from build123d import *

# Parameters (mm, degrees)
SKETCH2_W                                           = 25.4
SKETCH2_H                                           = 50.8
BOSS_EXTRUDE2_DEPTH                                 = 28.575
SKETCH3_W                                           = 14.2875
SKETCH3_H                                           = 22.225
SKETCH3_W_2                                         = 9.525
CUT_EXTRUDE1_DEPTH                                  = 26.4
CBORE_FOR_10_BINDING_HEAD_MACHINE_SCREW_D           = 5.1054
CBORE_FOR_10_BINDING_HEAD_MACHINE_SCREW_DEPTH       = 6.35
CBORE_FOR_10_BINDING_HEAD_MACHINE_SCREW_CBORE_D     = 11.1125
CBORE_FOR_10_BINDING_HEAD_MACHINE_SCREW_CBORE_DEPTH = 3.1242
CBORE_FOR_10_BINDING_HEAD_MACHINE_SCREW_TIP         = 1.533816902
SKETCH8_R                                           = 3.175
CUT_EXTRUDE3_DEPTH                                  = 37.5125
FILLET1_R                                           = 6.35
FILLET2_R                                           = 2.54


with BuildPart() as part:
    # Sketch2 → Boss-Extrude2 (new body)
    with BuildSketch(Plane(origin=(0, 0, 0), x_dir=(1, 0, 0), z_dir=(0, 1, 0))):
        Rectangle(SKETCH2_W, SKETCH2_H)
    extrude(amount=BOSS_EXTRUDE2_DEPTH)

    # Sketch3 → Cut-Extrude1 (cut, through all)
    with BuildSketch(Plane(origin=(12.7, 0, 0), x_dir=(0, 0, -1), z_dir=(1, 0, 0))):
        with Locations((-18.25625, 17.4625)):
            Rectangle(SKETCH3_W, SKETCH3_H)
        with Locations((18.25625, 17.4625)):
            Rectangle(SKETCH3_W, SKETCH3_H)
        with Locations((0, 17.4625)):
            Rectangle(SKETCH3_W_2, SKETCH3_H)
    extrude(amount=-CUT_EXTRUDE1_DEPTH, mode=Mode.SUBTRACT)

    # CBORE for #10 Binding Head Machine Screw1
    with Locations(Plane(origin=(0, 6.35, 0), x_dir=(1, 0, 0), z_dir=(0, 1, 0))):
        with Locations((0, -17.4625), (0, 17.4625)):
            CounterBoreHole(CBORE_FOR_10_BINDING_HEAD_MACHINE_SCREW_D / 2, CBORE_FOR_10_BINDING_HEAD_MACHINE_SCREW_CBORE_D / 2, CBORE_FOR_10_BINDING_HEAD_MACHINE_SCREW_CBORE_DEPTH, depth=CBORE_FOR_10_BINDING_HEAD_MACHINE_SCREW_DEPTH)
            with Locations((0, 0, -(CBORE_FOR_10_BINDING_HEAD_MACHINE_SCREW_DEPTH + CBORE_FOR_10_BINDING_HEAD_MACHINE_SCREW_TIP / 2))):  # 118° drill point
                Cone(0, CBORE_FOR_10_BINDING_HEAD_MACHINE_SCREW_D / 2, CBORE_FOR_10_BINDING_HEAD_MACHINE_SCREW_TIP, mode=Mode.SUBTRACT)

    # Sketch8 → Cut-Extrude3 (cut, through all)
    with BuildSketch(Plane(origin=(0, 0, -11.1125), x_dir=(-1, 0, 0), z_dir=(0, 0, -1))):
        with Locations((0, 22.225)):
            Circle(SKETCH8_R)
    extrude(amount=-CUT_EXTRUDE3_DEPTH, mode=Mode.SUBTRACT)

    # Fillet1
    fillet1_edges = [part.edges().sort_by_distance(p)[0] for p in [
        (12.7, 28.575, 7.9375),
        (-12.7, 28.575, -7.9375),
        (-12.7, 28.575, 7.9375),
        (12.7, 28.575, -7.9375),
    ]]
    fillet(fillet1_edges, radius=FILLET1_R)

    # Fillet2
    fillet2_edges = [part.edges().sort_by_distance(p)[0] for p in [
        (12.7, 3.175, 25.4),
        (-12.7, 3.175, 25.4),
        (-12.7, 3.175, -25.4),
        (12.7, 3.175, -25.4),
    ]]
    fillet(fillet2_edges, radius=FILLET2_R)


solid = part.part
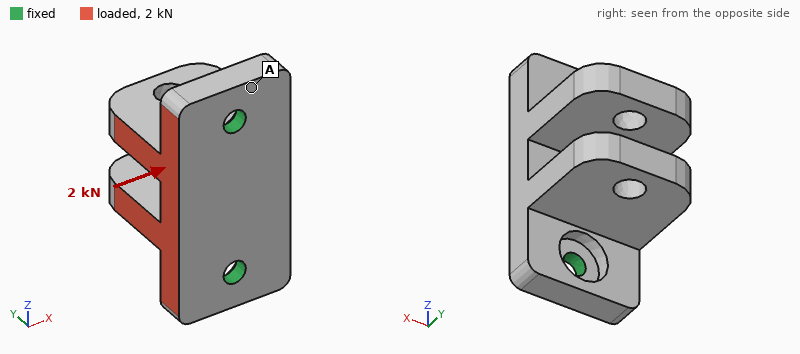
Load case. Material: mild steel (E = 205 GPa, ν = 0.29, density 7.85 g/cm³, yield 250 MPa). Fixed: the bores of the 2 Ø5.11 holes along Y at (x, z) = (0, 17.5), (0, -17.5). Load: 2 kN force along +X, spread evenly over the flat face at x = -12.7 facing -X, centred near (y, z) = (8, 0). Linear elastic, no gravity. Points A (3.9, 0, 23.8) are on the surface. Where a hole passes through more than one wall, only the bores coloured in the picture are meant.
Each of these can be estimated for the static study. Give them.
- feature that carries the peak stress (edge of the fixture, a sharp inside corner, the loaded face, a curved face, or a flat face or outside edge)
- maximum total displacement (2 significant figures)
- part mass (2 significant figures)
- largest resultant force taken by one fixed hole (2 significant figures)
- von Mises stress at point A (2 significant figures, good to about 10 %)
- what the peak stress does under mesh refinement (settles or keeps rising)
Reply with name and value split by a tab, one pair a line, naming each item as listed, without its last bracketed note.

feature that carries the peak stress	edge of the fixture
maximum total displacement	24 µm
part mass	110 g
largest resultant force taken by one fixed hole	1.0 kN
von Mises stress at point A	23 MPa
what the peak stress does under mesh refinement	keeps rising
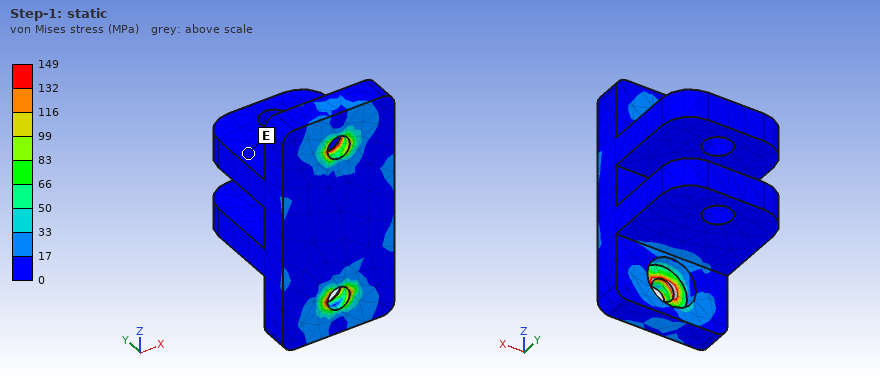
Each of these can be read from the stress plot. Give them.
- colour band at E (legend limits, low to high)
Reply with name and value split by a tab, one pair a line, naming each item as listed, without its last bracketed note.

colour band at E	0 to 17 MPa
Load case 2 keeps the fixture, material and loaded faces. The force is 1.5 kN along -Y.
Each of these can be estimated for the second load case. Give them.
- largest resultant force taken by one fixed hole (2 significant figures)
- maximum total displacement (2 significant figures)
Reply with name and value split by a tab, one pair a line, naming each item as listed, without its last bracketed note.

largest resultant force taken by one fixed hole	850 N
maximum total displacement	34 µm
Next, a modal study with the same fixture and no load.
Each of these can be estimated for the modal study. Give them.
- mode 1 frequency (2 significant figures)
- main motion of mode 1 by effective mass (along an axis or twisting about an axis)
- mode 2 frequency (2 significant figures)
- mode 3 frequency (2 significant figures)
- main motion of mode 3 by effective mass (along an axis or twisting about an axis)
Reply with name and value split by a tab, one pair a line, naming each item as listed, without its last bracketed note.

mode 1 frequency	4400 Hz
main motion of mode 1 by effective mass	along X
mode 2 frequency	6700 Hz
mode 3 frequency	8600 Hz
main motion of mode 3 by effective mass	along Z
